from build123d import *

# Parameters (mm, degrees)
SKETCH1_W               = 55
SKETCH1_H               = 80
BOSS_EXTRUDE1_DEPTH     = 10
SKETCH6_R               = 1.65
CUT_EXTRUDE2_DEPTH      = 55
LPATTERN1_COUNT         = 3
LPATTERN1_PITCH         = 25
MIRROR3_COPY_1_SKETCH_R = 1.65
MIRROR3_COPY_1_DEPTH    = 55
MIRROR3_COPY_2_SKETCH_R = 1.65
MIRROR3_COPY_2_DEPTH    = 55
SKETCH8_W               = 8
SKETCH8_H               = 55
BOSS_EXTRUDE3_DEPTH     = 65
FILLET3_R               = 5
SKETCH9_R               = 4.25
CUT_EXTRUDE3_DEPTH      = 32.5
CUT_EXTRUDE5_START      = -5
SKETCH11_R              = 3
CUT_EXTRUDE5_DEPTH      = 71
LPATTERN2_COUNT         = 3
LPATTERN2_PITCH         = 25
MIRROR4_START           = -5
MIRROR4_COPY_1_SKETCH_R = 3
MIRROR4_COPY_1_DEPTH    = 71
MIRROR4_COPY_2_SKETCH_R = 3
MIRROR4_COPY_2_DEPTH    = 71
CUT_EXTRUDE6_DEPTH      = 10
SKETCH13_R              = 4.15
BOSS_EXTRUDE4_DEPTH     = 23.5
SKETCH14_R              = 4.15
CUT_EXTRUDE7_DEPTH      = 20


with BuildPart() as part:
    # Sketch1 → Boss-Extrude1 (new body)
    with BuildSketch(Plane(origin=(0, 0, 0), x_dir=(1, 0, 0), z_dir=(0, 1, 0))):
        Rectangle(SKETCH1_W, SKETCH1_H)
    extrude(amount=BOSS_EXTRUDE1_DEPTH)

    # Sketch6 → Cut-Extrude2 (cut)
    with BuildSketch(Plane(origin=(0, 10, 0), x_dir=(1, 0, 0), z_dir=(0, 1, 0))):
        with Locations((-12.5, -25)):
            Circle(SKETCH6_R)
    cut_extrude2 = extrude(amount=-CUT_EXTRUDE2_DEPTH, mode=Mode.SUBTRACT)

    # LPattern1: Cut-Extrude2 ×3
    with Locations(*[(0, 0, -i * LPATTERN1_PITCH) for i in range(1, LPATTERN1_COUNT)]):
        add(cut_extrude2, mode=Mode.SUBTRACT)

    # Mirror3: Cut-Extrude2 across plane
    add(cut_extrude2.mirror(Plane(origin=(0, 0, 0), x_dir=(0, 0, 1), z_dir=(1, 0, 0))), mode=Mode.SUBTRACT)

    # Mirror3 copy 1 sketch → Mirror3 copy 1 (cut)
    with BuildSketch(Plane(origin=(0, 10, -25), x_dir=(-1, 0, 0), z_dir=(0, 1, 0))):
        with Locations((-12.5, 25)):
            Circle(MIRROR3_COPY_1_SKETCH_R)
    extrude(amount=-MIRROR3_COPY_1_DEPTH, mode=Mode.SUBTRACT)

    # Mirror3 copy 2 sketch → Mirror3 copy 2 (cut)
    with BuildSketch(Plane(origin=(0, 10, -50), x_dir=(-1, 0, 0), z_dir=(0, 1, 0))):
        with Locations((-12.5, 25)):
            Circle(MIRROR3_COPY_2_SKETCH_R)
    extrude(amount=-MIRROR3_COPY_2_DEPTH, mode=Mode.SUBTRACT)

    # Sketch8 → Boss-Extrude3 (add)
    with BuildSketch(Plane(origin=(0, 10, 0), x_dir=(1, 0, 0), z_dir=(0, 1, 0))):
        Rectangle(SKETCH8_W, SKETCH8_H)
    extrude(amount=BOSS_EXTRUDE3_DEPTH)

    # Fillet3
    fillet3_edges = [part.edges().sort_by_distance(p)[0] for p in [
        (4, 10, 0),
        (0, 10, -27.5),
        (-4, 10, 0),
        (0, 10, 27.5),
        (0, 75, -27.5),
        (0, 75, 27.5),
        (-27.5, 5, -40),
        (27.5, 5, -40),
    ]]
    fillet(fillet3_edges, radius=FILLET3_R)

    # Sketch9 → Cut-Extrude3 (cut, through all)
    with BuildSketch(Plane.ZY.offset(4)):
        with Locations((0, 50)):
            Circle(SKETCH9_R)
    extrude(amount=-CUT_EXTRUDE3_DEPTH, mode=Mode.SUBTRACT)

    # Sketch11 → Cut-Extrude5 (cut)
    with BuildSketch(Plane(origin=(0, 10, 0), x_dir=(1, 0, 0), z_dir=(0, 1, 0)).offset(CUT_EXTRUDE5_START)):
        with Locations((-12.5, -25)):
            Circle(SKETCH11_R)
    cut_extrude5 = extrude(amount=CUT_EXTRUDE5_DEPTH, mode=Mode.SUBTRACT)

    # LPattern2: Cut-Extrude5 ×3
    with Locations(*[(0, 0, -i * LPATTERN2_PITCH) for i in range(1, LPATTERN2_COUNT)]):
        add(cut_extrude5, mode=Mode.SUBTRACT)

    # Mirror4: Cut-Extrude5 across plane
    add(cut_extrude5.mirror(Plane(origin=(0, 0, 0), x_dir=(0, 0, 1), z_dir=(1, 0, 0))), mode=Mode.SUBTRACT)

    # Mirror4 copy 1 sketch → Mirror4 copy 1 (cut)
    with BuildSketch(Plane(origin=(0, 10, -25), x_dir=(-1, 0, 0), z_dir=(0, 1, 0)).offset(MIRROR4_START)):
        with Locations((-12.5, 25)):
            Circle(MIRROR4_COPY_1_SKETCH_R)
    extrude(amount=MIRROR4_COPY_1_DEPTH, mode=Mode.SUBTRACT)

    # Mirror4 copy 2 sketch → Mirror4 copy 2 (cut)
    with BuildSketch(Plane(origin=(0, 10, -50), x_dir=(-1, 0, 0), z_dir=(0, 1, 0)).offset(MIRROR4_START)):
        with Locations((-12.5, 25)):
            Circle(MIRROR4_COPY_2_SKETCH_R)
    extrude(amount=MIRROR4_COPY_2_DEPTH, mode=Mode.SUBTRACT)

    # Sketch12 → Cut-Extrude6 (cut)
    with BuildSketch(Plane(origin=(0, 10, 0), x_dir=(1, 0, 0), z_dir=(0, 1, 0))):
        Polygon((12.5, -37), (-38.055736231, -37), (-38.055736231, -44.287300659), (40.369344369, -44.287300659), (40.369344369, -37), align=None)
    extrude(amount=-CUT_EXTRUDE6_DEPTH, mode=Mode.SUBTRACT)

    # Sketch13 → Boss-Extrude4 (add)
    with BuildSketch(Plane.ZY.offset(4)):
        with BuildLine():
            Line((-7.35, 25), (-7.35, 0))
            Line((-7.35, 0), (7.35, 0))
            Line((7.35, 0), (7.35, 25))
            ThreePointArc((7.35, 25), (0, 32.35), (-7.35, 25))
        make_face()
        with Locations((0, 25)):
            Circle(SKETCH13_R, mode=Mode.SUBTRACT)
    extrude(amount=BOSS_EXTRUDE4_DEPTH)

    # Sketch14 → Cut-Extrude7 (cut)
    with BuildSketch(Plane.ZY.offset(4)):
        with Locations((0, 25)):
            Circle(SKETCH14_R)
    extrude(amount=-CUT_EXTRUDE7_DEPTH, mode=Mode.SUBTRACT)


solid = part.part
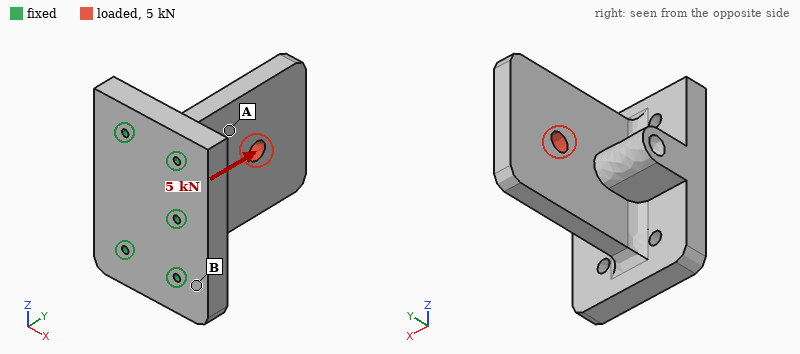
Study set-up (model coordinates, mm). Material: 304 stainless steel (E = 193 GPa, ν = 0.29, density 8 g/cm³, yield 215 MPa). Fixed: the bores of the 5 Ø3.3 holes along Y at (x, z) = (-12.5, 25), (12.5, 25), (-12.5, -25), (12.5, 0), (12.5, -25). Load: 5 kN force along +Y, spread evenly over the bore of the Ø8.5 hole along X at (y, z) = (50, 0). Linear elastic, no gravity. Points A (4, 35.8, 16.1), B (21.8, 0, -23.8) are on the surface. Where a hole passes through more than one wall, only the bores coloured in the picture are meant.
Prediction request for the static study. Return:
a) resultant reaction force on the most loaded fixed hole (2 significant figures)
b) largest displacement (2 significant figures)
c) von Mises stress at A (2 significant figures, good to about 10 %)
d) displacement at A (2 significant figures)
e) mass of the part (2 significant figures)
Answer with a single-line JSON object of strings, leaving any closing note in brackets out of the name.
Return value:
{"resultant reaction force on the most loaded fixed hole": "1.3 kN", "largest displacement": "5.9 µm", "von Mises stress at A": "12 MPa", "displacement at A": "3.3 µm", "mass of the part": "600 g"}
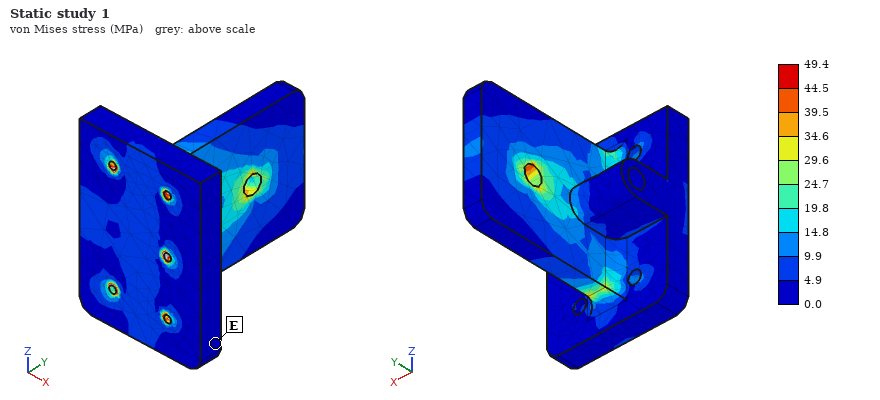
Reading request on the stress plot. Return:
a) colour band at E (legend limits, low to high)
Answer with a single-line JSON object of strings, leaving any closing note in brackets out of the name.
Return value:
{"colour band at E": "0.0 to 4.9 MPa"}
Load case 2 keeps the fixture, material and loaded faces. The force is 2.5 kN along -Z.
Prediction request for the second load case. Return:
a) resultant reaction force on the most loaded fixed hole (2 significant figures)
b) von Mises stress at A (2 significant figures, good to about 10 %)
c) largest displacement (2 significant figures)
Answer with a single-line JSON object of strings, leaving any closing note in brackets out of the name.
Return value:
{"resultant reaction force on the most loaded fixed hole": "1.4 kN", "von Mises stress at A": "12 MPa", "largest displacement": "14 µm"}
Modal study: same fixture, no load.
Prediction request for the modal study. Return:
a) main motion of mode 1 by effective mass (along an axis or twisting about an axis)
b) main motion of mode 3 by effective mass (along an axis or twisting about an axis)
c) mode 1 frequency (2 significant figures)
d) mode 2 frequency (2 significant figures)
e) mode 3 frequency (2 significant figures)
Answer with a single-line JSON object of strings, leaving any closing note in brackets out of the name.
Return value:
{"main motion of mode 1 by effective mass": "along X", "main motion of mode 3 by effective mass": "along Z", "mode 1 frequency": "1900 Hz", "mode 2 frequency": "4100 Hz", "mode 3 frequency": "5800 Hz"}
